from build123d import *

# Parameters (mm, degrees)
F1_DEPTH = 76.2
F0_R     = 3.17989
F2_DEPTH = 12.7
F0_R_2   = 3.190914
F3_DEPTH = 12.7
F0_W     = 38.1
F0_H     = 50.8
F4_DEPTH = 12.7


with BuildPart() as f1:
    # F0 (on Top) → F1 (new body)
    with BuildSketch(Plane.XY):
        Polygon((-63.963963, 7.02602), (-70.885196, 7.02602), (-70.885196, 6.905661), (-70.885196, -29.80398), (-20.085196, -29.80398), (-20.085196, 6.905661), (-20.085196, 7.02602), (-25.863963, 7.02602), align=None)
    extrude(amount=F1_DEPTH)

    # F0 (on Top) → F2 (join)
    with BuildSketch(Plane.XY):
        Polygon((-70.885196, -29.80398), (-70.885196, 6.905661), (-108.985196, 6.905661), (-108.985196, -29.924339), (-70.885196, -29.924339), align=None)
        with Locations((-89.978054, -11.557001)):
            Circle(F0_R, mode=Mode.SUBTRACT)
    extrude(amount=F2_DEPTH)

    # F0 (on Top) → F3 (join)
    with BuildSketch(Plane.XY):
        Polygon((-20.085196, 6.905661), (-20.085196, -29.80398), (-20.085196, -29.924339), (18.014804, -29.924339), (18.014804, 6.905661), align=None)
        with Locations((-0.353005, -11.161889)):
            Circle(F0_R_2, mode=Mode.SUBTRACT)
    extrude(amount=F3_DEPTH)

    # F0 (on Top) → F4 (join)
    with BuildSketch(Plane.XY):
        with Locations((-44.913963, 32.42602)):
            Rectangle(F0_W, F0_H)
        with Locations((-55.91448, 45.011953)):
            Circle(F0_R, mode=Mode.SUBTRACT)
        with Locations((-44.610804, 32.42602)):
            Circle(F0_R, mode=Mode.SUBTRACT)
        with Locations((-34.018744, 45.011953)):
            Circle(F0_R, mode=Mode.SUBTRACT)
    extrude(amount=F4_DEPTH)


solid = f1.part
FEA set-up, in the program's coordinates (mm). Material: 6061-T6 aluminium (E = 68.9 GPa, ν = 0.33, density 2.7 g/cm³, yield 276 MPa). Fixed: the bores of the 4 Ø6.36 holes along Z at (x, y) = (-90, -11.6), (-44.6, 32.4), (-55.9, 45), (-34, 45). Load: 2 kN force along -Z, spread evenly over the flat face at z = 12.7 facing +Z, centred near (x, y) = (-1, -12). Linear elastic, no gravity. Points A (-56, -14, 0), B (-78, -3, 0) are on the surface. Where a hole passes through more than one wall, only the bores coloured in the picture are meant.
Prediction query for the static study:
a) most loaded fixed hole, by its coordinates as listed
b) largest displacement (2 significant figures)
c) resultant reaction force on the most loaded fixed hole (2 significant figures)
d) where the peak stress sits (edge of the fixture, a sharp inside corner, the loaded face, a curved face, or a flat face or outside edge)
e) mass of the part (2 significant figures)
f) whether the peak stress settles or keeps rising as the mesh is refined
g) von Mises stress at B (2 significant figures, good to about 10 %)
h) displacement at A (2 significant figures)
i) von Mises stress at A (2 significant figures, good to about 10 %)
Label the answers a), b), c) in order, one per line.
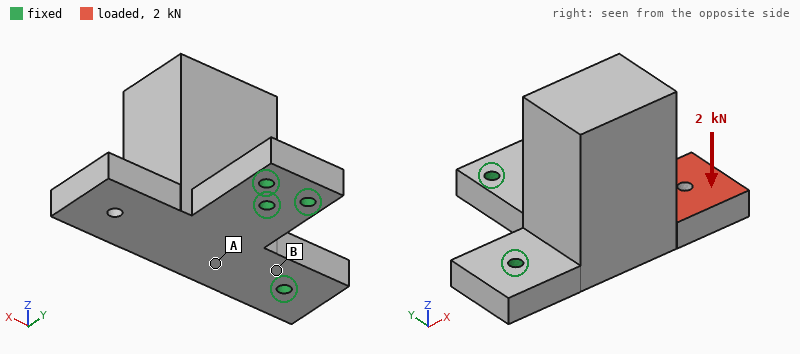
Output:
a) (-44.6, 32.4)
b) 0.32 mm
c) 3.1 kN
d) edge of the fixture
e) 540 g
f) keeps rising
g) 38 MPa
h) 0.055 mm
i) 14 MPa
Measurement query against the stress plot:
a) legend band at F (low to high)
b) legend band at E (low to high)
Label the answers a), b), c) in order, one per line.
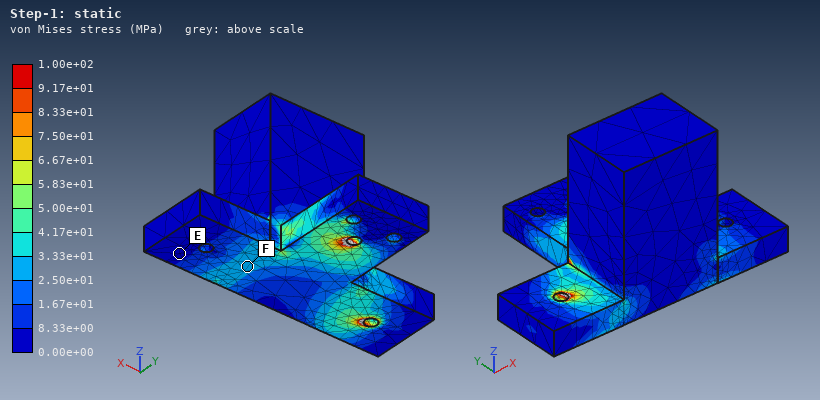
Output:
a) 2.50e+01 to 3.33e+01 MPa
b) 0.00e+00 to 8.33e+00 MPa
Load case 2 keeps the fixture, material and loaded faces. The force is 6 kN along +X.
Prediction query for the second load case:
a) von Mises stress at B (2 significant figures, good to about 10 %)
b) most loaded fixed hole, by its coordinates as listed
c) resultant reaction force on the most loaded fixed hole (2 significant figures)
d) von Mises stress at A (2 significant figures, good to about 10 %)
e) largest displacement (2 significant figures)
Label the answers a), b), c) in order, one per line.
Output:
a) 6.7 MPa
b) (-90, -11.6)
c) 5.0 kN
d) 8.6 MPa
e) 0.12 mm
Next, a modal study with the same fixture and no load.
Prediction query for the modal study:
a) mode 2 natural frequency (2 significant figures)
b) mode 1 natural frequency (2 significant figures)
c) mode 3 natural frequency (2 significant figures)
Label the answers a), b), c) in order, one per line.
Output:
a) 2200 Hz
b) 970 Hz
c) 4400 Hz
